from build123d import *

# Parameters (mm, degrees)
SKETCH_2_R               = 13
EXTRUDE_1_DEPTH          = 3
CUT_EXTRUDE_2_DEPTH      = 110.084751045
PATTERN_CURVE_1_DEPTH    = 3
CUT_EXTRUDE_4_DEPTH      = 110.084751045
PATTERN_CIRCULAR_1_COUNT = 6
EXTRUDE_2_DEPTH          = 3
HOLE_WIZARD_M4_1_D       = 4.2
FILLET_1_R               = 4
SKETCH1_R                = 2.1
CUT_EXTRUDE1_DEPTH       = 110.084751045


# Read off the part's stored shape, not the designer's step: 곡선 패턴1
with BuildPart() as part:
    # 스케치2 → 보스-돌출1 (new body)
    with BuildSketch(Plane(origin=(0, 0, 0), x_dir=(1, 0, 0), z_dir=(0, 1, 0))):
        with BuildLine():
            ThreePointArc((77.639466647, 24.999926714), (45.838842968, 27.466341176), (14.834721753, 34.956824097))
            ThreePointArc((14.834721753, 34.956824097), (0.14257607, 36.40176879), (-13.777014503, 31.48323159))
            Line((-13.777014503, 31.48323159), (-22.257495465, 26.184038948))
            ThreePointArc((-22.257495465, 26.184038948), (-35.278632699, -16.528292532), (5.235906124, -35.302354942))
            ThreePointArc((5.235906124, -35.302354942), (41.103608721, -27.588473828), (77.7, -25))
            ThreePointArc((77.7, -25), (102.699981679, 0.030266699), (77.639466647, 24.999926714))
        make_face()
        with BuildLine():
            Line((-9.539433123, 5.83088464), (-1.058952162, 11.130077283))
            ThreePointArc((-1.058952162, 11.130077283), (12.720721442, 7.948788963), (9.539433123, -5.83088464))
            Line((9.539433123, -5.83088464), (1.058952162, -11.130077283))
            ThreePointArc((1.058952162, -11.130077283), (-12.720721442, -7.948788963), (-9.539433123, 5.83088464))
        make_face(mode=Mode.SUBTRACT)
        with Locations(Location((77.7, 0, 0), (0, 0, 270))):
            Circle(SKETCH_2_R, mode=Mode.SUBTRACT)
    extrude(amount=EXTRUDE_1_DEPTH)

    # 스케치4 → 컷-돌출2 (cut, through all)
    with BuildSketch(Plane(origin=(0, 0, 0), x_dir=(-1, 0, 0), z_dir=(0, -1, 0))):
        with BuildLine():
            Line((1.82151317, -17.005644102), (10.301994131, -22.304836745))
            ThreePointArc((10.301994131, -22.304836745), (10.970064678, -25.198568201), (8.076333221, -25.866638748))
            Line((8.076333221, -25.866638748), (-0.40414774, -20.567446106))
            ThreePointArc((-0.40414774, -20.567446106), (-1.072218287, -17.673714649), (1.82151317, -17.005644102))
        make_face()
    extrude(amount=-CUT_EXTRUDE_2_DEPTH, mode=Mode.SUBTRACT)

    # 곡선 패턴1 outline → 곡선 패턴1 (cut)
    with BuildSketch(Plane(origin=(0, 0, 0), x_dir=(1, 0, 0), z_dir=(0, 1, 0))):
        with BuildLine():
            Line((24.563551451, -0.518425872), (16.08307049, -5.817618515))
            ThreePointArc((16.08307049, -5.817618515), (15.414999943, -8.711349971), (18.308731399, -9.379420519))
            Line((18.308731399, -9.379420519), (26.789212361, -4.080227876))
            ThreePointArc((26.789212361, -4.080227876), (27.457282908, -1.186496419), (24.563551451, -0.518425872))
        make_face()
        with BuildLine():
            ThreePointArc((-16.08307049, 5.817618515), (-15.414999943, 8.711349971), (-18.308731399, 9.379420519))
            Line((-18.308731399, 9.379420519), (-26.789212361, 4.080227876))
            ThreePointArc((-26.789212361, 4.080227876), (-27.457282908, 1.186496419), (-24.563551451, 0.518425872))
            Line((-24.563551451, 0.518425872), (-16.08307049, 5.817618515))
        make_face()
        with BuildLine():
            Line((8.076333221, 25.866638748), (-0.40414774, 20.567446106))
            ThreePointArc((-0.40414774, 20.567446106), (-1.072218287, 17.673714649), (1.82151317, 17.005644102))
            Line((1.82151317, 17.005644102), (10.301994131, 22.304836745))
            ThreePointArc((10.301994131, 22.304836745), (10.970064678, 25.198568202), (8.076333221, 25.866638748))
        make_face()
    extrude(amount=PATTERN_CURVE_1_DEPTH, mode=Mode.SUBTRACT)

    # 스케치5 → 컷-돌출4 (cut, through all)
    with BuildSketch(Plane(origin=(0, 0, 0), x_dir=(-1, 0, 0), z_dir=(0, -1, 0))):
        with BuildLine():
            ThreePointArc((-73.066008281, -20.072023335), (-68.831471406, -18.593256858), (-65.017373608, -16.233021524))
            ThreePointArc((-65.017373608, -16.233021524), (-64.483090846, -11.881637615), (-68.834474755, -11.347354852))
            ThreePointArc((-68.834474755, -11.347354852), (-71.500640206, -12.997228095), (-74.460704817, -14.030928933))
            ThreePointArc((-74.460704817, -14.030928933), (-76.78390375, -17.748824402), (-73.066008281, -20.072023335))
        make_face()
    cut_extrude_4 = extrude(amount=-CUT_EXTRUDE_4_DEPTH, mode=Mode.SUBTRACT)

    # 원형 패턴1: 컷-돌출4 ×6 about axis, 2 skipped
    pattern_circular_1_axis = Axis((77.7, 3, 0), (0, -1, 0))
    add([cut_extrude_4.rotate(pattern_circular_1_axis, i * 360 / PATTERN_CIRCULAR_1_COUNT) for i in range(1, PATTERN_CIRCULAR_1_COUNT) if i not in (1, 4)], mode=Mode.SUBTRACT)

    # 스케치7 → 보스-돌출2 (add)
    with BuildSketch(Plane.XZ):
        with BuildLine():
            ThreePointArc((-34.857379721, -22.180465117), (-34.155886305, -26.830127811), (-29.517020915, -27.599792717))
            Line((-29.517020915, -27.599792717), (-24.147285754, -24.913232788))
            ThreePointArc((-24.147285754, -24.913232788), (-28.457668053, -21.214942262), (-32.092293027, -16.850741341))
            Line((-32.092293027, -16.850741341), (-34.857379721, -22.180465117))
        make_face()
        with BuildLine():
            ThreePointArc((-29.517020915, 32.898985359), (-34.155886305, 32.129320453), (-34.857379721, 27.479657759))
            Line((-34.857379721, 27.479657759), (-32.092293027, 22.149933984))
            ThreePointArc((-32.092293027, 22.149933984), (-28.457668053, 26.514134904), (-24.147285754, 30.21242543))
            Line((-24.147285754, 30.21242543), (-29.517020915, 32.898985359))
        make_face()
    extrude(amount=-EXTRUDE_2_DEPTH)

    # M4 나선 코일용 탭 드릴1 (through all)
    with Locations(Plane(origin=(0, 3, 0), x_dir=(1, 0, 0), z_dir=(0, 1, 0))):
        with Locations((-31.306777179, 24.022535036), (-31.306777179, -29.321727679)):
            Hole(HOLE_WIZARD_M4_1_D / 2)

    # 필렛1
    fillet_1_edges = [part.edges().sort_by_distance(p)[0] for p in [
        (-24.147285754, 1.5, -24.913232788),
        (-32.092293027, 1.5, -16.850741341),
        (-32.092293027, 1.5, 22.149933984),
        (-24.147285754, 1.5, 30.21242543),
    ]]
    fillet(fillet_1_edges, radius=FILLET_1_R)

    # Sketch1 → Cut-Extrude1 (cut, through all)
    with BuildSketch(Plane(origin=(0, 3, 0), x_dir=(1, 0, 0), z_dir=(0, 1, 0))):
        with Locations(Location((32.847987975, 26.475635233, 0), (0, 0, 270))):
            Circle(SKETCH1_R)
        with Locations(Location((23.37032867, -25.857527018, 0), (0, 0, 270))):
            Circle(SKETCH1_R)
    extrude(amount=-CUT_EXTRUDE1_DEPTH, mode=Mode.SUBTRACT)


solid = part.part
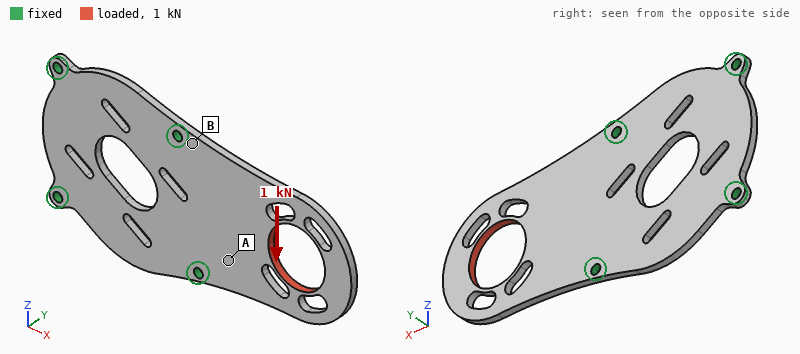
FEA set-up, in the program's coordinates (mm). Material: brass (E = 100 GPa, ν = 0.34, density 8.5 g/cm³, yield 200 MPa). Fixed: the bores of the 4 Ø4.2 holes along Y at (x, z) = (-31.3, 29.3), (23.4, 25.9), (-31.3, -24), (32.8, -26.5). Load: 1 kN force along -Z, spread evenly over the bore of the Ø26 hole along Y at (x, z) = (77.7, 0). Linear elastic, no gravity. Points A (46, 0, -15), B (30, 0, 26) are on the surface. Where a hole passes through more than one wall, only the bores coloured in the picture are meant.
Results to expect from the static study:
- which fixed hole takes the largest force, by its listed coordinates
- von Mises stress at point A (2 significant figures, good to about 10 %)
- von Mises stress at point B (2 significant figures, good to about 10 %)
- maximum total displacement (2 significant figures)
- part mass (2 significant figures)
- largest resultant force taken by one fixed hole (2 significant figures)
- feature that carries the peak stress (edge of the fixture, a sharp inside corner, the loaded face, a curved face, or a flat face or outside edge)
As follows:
(32.8, -26.5)
14 MPa
29 MPa
67 µm
160 g
1.1 kN
a curved face
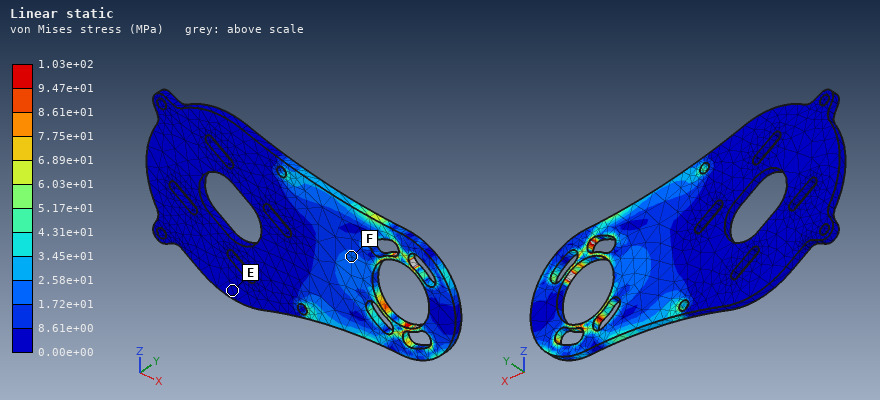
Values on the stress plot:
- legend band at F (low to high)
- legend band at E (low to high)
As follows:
1.72e+01 to 2.58e+01 MPa
0.00e+00 to 8.61e+00 MPa
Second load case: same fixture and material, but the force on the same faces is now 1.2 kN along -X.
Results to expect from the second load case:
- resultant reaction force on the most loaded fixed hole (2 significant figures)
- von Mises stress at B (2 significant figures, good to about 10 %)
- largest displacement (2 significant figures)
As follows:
570 N
16 MPa
23 µm
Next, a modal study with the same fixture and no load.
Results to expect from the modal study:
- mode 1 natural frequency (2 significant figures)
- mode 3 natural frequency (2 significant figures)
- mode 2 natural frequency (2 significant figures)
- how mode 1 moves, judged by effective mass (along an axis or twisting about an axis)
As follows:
390 Hz
1500 Hz
1200 Hz
along Y
